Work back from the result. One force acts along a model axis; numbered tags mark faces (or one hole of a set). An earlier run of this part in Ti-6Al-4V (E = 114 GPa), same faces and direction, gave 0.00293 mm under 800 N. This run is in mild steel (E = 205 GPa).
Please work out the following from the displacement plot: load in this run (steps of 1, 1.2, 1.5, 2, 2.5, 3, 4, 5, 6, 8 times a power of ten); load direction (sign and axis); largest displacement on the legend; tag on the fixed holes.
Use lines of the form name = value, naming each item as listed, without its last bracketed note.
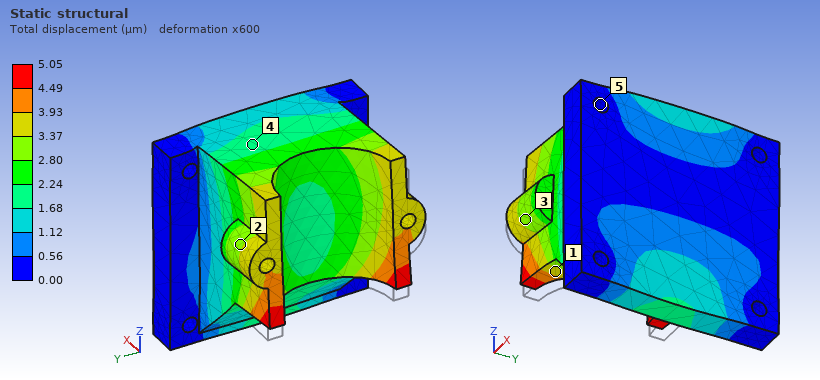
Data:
load in this run = 2.5 kN
load direction = +Z
largest displacement on the legend = 5.05 µm
tag on the fixed holes = 5
